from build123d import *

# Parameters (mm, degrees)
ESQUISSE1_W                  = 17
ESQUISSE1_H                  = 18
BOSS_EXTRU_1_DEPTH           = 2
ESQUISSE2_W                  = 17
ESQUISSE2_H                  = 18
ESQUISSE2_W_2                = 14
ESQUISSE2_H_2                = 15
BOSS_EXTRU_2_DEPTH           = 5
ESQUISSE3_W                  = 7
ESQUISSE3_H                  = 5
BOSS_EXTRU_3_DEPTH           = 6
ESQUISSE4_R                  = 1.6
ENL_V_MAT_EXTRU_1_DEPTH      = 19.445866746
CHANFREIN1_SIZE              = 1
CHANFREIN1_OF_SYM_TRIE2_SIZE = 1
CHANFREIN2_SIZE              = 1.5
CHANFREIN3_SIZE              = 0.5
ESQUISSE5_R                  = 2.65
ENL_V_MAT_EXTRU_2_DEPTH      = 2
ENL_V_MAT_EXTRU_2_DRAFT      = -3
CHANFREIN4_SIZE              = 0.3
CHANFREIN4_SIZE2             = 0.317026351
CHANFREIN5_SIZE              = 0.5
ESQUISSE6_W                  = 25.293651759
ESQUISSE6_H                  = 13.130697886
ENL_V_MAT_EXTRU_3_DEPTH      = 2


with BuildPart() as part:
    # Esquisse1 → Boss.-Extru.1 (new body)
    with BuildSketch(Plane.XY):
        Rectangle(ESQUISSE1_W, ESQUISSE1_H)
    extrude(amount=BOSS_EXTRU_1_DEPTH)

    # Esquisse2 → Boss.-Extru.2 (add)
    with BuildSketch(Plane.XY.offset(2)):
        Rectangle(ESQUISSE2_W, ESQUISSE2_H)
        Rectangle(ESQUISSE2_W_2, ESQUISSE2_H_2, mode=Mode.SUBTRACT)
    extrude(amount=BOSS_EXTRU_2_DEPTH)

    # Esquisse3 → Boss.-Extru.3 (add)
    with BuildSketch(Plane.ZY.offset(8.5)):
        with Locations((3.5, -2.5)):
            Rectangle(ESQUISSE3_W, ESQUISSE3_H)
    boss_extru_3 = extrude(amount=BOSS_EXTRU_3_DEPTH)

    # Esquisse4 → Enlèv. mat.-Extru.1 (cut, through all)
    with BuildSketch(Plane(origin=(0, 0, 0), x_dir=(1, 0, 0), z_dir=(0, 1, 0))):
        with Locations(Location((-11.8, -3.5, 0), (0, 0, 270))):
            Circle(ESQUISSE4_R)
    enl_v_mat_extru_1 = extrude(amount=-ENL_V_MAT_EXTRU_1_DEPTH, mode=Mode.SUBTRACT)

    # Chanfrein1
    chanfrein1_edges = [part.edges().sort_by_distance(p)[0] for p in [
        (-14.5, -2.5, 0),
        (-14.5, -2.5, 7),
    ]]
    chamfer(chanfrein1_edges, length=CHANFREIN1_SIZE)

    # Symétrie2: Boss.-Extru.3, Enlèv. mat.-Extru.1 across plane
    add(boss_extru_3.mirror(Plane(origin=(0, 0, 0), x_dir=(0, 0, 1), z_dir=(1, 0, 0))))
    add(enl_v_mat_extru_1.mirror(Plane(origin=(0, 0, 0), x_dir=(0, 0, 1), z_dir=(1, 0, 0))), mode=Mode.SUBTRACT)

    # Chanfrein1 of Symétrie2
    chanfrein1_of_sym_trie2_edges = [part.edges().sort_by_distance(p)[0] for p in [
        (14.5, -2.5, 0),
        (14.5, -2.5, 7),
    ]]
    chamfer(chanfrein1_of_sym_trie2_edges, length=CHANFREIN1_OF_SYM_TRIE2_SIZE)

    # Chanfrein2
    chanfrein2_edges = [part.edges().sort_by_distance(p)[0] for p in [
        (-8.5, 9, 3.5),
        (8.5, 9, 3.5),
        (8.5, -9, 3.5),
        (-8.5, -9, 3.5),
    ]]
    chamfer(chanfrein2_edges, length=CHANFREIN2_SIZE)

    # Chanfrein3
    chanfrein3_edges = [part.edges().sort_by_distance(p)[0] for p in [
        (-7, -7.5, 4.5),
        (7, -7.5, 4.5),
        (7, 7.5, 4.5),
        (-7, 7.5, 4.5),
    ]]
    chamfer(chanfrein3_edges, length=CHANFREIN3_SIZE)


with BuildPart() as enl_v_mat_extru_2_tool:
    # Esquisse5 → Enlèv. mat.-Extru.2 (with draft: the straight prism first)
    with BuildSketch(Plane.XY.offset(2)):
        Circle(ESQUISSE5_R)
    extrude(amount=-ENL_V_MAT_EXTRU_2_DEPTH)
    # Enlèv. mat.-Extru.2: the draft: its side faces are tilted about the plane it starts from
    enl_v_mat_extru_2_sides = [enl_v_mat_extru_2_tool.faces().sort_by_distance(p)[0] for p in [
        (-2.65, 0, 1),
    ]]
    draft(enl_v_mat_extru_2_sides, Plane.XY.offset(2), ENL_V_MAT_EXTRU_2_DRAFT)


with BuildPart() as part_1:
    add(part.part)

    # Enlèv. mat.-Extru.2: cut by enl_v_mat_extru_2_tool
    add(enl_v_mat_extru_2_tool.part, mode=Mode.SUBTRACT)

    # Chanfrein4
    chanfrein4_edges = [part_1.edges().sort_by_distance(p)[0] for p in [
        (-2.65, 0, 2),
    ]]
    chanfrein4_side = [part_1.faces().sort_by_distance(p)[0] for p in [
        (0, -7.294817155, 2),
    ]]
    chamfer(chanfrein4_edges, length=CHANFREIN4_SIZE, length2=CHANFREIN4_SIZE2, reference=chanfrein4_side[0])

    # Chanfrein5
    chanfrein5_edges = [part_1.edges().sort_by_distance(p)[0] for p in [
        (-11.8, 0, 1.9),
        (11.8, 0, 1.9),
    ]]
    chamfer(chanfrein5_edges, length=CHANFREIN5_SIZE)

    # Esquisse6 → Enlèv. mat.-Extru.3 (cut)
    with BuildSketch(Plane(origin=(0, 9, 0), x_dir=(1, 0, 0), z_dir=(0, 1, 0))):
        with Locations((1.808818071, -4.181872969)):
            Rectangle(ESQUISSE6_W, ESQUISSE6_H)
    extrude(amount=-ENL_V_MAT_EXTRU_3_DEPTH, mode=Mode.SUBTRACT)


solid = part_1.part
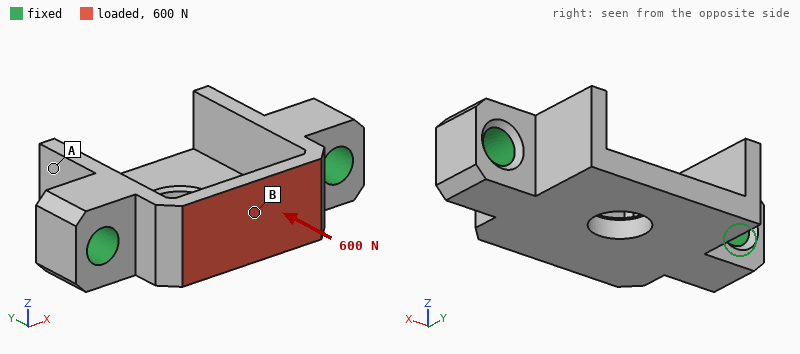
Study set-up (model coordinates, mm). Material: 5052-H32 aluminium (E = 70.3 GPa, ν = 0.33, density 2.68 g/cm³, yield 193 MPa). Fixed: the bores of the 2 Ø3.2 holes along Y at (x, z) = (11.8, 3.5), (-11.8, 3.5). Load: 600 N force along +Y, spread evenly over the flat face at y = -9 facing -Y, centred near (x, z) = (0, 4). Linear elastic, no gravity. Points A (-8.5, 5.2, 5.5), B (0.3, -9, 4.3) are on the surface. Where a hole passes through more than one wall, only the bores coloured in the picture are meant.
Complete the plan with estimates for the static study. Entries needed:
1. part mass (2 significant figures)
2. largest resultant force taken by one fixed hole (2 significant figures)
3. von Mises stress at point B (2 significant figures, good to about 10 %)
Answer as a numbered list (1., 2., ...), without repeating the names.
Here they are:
1. 3.1 g
2. 330 N
3. 52 MPa
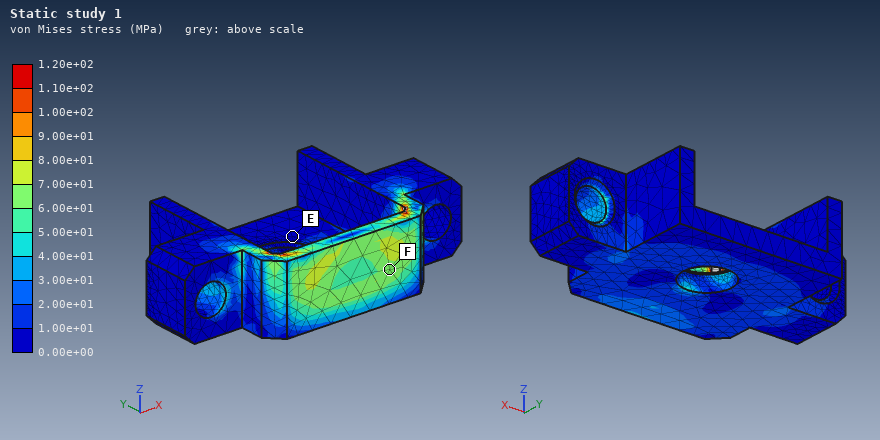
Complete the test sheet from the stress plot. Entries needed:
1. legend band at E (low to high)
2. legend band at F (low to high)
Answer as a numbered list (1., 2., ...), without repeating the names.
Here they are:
1. 0.00e+00 to 1.00e+01 MPa
2. 6.00e+01 to 7.00e+01 MPa
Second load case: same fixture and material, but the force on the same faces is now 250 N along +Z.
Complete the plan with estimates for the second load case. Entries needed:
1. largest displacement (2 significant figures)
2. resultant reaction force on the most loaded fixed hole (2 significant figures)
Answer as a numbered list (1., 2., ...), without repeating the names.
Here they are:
1. 16 µm
2. 140 N
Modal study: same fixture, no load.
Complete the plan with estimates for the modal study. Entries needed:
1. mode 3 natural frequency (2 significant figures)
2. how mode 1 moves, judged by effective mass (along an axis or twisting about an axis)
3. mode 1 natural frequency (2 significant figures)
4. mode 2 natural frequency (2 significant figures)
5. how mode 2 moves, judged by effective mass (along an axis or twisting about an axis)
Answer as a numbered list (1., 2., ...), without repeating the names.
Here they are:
1. 35 kHz
2. along Z
3. 23 kHz
4. 32 kHz
5. along Z
